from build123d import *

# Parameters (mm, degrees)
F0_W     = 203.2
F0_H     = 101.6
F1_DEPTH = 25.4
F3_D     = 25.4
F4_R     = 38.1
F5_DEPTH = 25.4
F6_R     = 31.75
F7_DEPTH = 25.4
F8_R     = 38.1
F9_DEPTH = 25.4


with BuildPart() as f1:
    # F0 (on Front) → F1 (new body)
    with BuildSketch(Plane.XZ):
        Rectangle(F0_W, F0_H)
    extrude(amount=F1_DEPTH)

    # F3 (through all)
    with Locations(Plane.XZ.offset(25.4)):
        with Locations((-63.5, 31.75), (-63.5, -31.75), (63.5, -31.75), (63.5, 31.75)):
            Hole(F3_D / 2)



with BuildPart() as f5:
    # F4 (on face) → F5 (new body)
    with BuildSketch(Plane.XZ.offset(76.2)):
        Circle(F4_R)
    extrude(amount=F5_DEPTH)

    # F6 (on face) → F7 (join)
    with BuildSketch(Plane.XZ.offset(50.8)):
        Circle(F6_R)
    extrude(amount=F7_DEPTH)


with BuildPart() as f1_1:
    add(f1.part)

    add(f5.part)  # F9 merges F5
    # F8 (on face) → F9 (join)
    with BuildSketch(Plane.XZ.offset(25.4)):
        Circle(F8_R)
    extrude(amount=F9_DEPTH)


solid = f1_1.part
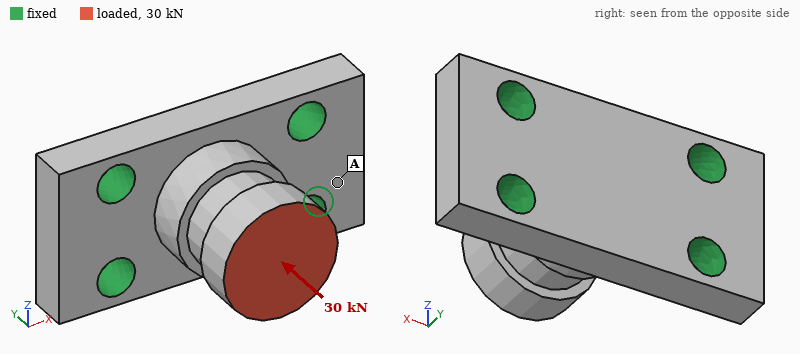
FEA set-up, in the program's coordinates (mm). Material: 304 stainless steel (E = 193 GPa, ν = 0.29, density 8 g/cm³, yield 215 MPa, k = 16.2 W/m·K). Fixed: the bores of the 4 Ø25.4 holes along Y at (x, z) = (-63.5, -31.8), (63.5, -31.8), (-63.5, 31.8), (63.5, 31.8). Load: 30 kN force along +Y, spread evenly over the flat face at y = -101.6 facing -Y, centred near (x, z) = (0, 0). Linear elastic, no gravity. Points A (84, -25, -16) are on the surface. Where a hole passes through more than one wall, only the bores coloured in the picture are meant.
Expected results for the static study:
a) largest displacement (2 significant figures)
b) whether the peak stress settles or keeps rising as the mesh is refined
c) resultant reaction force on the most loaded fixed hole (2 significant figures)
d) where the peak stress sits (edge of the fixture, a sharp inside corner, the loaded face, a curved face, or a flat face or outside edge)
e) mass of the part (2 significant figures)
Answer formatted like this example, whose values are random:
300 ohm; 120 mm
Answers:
8.8 µm; keeps rising; 7.9 kN; edge of the fixture; 6.3 kg
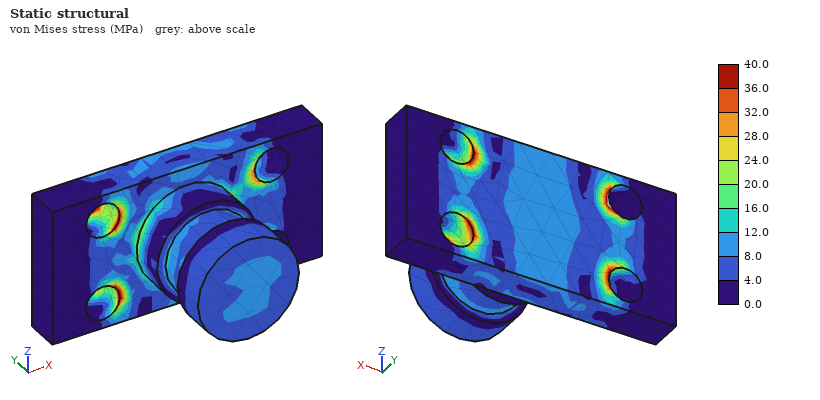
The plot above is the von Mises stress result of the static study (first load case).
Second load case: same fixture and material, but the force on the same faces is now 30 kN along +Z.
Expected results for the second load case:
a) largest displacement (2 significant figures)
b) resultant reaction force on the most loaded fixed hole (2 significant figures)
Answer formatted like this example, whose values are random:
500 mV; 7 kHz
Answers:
86 µm; 22 kN
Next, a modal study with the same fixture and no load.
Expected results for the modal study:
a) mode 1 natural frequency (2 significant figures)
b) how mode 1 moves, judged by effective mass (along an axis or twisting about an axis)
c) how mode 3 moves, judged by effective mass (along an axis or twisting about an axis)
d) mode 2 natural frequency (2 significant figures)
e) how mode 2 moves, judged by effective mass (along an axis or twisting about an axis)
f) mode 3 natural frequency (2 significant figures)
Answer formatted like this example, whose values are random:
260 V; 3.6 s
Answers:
3100 Hz; along Z; along Y; 4200 Hz; along X; 5700 Hz
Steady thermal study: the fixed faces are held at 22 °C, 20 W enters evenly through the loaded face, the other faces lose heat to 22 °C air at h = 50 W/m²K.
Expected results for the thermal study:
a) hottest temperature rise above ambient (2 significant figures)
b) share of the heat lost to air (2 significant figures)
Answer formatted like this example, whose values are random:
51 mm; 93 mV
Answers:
20 K; 65 %
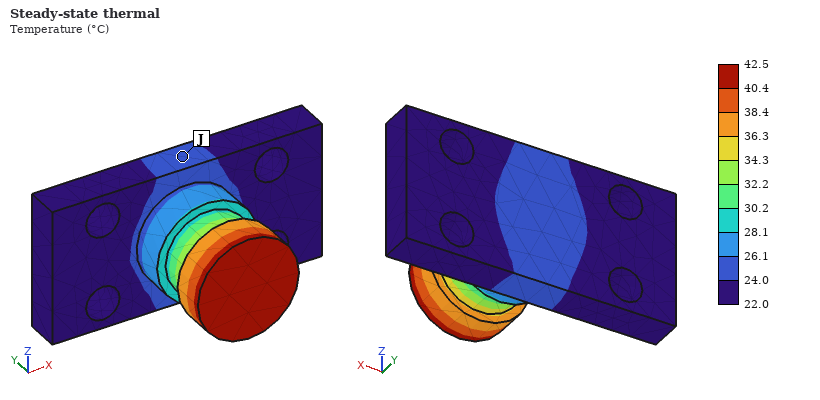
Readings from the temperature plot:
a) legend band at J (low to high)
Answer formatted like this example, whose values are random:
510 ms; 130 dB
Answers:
24.0 to 26.1 °C
